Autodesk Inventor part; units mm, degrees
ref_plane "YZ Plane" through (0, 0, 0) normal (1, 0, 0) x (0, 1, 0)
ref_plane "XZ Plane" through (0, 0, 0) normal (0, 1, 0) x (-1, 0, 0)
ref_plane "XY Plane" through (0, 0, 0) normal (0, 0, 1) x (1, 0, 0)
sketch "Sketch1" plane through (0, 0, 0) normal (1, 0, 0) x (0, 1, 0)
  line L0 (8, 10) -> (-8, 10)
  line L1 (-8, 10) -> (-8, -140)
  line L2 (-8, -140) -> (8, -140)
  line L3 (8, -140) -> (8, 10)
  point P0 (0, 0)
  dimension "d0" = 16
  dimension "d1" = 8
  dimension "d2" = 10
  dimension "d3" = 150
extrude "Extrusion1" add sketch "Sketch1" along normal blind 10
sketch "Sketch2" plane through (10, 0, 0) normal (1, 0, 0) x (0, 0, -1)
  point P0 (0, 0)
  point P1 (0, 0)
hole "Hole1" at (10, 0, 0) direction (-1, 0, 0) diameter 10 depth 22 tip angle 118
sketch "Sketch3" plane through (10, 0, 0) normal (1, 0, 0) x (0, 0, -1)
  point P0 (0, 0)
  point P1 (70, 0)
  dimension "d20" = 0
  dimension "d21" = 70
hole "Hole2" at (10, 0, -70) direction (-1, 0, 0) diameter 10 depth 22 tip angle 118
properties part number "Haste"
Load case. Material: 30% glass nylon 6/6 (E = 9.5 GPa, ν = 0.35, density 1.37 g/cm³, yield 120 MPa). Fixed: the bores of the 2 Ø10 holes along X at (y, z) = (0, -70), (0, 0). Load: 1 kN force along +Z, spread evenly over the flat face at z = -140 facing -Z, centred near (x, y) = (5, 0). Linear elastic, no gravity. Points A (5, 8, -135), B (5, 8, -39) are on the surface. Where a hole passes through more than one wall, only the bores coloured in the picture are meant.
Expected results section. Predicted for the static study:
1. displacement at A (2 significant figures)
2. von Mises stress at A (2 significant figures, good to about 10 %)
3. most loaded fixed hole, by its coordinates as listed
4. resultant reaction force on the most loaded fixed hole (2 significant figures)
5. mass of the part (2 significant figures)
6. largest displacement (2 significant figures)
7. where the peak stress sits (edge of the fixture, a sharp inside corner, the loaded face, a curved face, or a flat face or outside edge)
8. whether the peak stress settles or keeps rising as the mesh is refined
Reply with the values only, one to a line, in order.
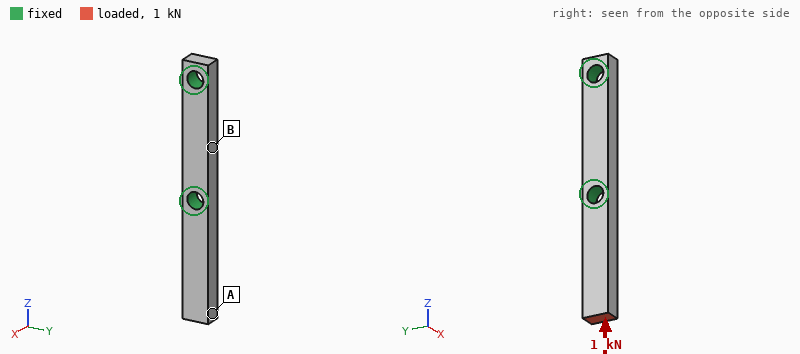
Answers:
41 µm
6.2 MPa
(0, -70)
1000 N
31 g
44 µm
edge of the fixture
keeps rising
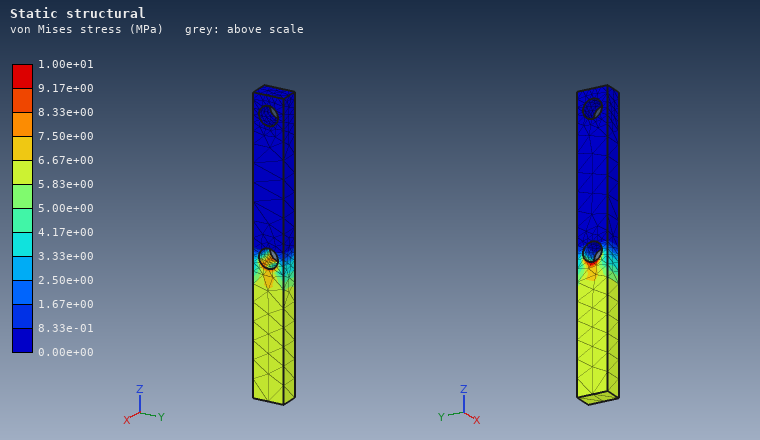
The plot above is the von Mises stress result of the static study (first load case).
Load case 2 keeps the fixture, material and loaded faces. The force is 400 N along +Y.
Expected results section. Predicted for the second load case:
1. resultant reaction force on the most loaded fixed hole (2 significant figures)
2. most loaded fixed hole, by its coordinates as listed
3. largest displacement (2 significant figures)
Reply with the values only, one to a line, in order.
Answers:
420 N
(0, -70)
1.4 mm
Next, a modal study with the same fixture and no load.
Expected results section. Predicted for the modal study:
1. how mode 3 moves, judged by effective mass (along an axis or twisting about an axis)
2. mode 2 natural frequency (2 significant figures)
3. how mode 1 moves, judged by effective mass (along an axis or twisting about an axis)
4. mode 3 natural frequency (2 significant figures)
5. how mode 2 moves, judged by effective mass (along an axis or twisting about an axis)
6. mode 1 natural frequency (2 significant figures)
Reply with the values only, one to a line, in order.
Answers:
twisting about Z
1400 Hz
along X
5100 Hz
along Y
950 Hz
